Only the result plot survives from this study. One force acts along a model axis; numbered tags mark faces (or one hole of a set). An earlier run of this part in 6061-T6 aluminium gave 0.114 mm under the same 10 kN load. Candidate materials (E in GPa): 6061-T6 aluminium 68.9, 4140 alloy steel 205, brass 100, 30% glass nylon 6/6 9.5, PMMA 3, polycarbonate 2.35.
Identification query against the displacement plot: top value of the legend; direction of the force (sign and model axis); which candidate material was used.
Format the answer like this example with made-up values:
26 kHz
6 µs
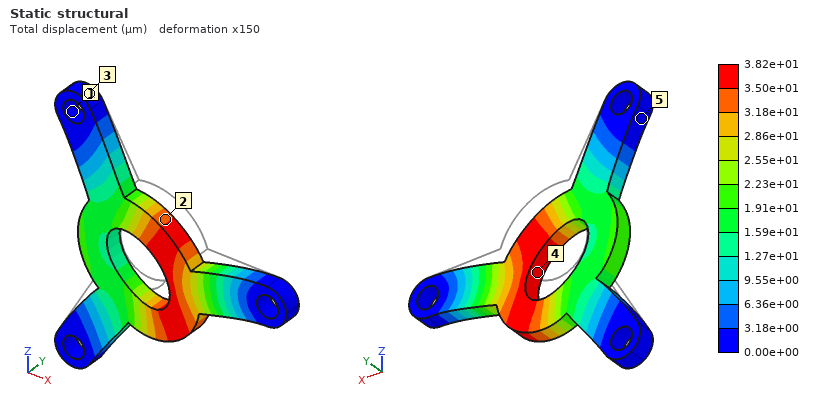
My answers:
3.82e+01 µm
-Z
4140 alloy steel
